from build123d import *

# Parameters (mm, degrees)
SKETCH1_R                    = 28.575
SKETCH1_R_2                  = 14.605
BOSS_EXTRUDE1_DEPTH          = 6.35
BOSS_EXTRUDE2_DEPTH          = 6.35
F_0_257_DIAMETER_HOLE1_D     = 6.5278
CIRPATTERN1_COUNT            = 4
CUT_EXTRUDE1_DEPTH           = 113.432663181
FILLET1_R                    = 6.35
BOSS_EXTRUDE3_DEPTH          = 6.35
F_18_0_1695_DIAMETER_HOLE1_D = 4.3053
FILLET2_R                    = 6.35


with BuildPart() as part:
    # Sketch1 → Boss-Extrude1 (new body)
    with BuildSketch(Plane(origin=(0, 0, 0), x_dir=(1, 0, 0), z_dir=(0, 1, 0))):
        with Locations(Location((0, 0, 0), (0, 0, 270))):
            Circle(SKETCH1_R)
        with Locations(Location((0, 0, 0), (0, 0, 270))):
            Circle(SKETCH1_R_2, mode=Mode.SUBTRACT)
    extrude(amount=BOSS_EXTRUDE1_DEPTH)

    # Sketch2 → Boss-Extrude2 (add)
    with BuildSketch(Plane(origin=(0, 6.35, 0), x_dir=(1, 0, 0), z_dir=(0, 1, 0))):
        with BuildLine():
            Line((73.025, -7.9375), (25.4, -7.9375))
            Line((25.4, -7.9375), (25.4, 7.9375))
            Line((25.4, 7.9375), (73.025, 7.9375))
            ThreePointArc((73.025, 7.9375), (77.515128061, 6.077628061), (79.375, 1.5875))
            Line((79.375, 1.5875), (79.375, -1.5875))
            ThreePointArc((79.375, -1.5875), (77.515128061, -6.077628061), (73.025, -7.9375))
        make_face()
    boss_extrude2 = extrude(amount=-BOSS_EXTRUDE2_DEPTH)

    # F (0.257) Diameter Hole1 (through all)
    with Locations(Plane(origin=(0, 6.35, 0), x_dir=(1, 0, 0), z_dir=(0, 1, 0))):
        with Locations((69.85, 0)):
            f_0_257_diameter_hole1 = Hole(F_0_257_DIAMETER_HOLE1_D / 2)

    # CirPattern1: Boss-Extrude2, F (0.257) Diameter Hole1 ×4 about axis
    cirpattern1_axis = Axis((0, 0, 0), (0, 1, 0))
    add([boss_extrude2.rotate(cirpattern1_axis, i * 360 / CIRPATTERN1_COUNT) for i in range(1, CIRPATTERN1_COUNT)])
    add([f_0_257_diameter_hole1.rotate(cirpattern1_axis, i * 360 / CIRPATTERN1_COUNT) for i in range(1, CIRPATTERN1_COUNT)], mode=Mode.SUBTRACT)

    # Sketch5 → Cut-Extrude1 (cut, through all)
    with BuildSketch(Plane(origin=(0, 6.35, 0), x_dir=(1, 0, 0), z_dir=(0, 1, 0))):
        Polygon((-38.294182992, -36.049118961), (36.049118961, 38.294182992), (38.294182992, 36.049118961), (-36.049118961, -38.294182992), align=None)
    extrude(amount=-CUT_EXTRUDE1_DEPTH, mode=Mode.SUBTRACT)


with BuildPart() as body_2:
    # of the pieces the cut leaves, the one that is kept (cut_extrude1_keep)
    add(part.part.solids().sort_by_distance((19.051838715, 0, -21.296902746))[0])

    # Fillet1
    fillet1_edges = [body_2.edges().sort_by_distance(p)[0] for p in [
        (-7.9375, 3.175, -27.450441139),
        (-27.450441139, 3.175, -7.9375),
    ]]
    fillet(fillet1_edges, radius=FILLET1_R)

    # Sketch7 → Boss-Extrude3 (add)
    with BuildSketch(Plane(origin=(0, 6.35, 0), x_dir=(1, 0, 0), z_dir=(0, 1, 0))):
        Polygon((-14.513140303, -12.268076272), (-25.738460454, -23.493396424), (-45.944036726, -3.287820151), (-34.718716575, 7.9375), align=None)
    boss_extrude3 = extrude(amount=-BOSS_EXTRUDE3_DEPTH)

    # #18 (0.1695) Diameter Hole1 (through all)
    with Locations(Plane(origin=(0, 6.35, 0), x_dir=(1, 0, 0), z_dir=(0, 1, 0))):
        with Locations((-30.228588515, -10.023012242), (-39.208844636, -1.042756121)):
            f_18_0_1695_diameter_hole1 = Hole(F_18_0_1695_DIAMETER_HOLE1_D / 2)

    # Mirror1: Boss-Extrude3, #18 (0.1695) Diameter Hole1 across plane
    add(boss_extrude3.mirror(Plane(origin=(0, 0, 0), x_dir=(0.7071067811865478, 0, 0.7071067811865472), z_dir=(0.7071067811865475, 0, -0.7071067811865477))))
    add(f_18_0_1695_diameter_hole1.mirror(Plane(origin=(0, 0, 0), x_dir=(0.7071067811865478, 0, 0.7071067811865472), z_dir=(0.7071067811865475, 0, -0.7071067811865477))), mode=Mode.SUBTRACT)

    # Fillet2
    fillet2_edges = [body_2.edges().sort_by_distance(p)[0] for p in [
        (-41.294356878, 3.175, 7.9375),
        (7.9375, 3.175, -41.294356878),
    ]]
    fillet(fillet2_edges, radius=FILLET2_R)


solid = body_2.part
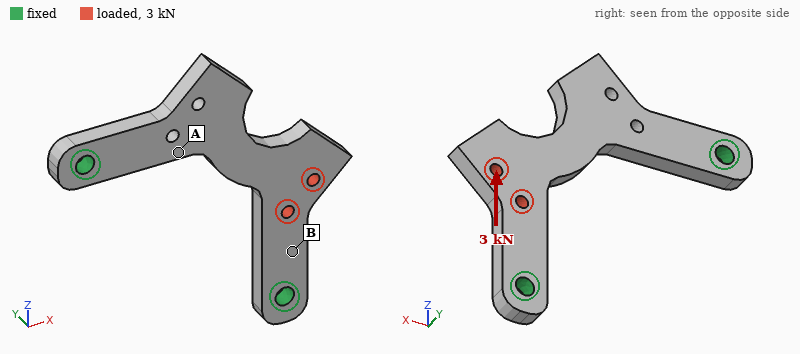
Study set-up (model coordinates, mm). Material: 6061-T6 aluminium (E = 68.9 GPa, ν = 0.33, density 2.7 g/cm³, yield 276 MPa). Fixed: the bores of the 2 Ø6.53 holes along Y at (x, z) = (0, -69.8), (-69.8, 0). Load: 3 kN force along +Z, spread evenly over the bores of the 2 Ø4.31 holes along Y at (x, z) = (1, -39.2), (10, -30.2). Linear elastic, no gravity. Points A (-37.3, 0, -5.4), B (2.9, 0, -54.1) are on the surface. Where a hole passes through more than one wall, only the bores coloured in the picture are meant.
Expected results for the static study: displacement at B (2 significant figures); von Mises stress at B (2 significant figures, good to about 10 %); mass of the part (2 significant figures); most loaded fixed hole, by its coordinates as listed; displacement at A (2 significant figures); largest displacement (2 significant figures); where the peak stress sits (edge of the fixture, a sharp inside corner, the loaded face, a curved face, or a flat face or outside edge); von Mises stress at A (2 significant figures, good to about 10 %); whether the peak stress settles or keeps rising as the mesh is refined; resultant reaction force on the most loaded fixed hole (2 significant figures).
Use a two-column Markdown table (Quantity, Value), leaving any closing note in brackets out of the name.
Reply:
| Quantity | Value |
|---|---|
| displacement at B | 7.2 µm |
| von Mises stress at B | 34 MPa |
| mass of the part | 46 g |
| most loaded fixed hole, by its coordinates as listed | (0, -69.8) |
| displacement at A | 7.2 µm |
| largest displacement | 25 µm |
| where the peak stress sits | edge of the fixture |
| von Mises stress at A | 7.7 MPa |
| whether the peak stress settles or keeps rising as the mesh is refined | keeps rising |
| resultant reaction force on the most loaded fixed hole | 2.9 kN |
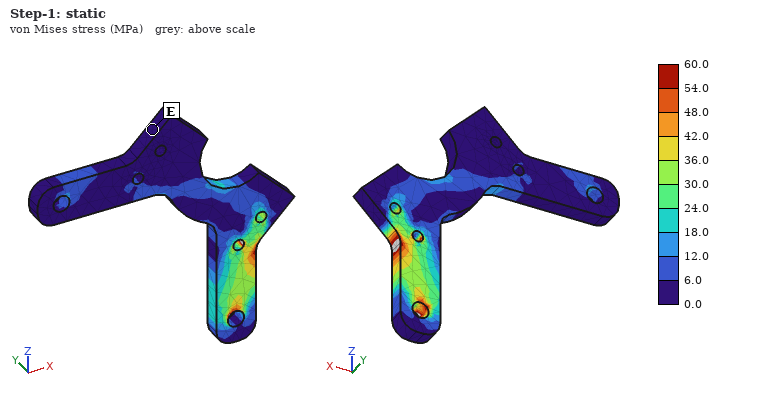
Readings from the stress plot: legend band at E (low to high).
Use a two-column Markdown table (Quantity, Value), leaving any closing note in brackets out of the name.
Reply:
| Quantity | Value |
|---|---|
| legend band at E | 0.0 to 6.0 MPa |
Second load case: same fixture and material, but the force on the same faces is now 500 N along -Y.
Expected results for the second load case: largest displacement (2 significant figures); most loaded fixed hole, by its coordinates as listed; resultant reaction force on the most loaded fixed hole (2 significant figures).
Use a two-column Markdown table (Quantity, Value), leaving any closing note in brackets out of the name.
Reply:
| Quantity | Value |
|---|---|
| largest displacement | 0.31 mm |
| most loaded fixed hole, by its coordinates as listed | (0, -69.8) |
| resultant reaction force on the most loaded fixed hole | 430 N |
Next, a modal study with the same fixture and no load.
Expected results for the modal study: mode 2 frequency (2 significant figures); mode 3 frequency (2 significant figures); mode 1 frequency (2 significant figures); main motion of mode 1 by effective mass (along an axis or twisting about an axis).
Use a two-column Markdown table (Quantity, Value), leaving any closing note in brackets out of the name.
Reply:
| Quantity | Value |
|---|---|
| mode 2 frequency | 3300 Hz |
| mode 3 frequency | 5600 Hz |
| mode 1 frequency | 1400 Hz |
| main motion of mode 1 by effective mass | along Y |
